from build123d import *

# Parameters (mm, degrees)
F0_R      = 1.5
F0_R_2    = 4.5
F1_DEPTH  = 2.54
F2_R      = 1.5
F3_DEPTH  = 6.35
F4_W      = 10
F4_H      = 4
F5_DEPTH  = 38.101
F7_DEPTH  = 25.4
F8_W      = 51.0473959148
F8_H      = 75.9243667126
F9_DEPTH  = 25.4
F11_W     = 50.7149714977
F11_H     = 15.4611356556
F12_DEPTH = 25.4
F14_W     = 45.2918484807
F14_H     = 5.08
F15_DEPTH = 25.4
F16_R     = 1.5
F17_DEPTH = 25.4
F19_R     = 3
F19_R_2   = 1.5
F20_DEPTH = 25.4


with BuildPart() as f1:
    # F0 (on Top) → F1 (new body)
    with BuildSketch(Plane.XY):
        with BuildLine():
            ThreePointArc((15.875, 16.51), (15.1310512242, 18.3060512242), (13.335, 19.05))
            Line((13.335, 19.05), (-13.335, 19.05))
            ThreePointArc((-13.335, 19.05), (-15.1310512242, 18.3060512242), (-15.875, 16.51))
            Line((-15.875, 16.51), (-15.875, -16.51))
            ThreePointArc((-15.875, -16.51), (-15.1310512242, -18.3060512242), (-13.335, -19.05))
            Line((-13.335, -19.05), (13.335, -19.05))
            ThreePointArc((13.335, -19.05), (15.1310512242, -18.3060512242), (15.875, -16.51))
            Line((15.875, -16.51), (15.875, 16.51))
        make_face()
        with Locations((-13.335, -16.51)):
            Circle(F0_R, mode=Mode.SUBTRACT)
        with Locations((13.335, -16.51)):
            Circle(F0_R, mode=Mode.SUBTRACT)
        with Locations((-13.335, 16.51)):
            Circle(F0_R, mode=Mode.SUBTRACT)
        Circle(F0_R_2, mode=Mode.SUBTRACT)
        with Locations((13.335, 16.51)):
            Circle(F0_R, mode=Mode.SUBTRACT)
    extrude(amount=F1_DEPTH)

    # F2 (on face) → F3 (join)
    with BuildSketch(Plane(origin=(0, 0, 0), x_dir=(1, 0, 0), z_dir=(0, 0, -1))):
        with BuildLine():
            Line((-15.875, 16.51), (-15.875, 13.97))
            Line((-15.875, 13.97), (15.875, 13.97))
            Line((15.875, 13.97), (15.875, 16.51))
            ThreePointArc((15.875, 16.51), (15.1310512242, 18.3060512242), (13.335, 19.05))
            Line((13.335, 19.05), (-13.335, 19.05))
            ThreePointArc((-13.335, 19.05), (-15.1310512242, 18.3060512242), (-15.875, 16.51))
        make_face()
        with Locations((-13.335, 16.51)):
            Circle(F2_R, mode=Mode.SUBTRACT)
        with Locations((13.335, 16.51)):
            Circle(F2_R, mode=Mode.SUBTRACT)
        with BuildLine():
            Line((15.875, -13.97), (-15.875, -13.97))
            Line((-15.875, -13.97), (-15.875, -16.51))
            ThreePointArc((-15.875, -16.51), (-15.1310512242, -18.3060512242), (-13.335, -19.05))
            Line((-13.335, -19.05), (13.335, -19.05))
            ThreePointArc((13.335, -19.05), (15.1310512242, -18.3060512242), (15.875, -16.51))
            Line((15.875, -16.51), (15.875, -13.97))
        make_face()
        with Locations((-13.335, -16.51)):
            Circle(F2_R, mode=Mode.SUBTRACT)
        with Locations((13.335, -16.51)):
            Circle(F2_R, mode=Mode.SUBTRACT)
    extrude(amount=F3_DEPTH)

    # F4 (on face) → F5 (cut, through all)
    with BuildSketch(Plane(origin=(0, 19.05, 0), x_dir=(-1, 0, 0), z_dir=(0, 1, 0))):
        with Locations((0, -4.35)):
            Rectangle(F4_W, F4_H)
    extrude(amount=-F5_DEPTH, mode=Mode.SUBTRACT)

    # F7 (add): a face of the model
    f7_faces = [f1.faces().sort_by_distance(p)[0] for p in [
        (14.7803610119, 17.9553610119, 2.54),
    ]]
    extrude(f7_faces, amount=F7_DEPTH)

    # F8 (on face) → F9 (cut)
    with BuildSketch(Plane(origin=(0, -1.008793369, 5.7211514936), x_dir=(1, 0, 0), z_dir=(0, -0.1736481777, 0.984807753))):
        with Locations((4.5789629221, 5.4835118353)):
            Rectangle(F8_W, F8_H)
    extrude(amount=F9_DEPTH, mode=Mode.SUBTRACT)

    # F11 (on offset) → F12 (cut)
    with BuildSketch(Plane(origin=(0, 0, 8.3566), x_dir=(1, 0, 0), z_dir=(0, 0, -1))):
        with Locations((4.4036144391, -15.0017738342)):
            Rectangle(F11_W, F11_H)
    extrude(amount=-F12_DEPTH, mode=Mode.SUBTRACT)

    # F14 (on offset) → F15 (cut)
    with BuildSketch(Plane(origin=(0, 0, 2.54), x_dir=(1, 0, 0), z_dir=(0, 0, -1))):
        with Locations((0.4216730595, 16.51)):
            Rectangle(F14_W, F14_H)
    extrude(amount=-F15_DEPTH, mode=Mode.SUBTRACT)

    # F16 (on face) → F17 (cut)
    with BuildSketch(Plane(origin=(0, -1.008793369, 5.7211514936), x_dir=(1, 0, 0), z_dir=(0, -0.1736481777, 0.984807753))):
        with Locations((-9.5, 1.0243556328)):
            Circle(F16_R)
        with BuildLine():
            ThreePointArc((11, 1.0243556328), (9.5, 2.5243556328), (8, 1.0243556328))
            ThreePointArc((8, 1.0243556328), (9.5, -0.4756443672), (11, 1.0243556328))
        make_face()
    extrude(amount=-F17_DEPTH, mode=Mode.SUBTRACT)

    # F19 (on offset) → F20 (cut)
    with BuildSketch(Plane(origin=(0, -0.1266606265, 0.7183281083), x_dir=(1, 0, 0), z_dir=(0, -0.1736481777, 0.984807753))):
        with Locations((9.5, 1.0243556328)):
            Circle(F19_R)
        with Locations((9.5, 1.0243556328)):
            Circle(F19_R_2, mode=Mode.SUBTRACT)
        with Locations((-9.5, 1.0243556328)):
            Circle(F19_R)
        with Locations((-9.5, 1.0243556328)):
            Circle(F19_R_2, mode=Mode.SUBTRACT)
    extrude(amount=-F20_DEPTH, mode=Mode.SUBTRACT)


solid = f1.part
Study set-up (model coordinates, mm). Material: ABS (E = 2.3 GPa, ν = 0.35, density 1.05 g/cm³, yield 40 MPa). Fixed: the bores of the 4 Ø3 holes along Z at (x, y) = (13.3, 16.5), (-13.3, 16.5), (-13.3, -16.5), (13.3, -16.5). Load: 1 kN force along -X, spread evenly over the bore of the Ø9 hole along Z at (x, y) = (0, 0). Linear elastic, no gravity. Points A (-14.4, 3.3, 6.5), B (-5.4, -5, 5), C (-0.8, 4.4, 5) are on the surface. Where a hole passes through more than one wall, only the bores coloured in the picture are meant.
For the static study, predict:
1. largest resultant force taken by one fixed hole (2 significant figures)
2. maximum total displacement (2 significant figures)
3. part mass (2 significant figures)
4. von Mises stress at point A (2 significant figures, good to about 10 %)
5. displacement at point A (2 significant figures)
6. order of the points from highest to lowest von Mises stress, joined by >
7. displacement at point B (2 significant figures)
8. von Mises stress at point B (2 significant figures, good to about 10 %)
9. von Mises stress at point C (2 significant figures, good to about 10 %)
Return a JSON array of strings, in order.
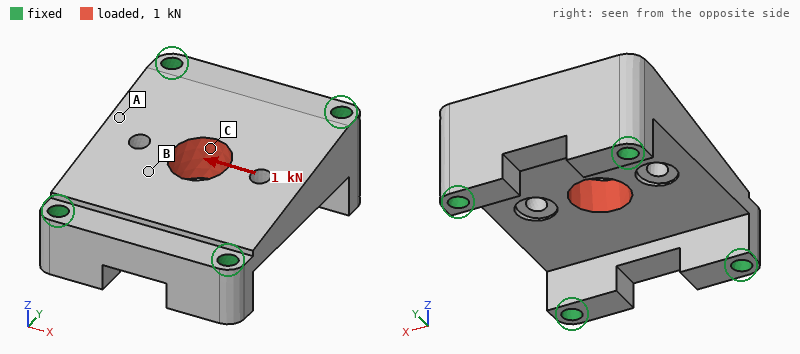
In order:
["370 N", "75 µm", "8.1 g", "2.0 MPa", "46 µm", "C > B > A", "58 µm", "5.3 MPa", "11 MPa"]
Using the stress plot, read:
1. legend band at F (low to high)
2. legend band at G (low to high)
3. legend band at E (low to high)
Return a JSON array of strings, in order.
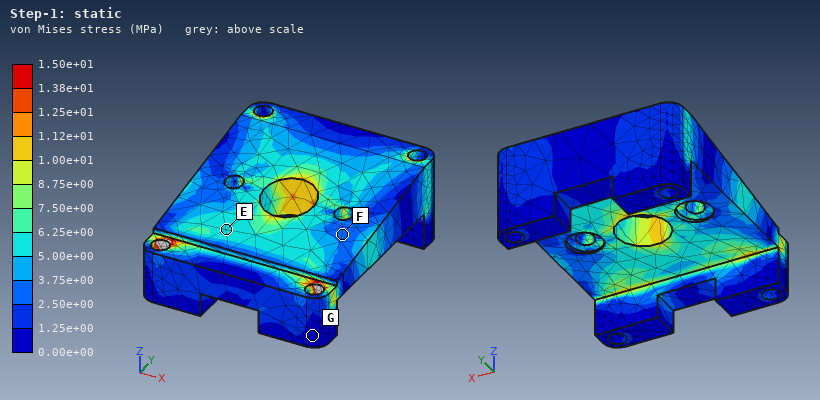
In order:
["2.50e+00 to 3.75e+00 MPa", "0.00e+00 to 1.25e+00 MPa", "5.00e+00 to 6.25e+00 MPa"]
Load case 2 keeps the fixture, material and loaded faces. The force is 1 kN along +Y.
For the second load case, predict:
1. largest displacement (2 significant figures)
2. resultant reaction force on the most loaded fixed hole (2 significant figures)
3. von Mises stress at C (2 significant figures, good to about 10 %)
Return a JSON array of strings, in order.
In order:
["85 µm", "370 N", "5.2 MPa"]
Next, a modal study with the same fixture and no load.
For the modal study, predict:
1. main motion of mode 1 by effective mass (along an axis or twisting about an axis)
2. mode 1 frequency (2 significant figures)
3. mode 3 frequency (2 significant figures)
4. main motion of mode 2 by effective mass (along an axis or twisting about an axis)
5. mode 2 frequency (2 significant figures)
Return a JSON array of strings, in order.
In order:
["along Z", "6100 Hz", "11 kHz", "twisting about Y", "8100 Hz"]
